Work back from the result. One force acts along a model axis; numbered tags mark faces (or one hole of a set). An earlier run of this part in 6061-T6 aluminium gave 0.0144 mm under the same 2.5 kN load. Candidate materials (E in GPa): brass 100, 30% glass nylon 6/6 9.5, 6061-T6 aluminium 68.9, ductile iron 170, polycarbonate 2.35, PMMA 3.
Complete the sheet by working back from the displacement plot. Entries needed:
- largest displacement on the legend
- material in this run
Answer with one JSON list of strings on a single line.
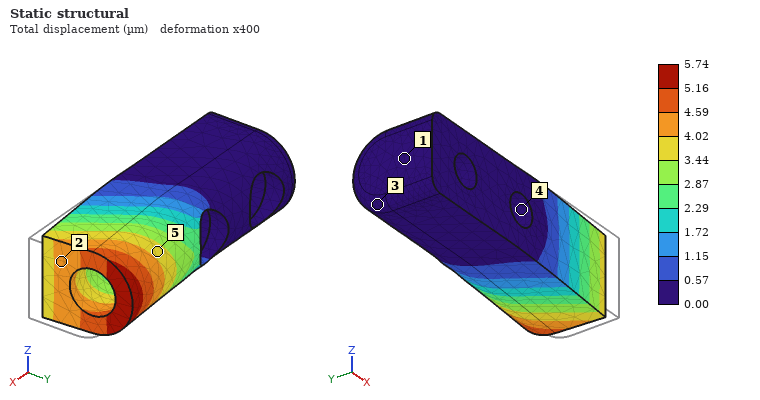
["5.74 µm", "ductile iron"]
